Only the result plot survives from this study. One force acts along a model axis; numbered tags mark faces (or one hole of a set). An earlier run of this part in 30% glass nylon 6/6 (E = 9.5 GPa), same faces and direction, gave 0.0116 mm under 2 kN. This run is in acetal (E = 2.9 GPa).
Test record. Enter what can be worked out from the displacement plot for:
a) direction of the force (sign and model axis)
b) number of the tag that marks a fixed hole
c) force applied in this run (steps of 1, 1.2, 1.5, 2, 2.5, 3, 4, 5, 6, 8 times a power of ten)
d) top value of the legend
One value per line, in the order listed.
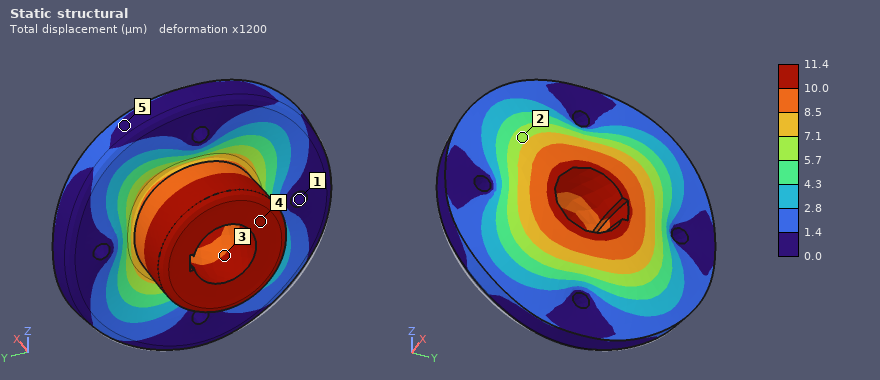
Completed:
+X
1
600 N
11.4 µm
